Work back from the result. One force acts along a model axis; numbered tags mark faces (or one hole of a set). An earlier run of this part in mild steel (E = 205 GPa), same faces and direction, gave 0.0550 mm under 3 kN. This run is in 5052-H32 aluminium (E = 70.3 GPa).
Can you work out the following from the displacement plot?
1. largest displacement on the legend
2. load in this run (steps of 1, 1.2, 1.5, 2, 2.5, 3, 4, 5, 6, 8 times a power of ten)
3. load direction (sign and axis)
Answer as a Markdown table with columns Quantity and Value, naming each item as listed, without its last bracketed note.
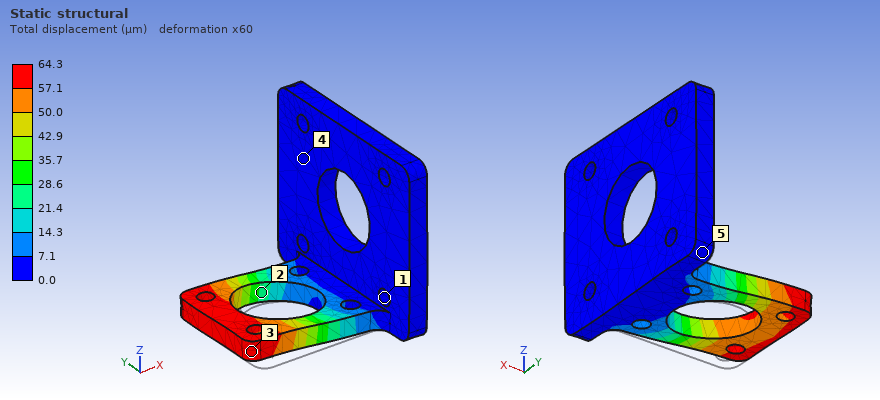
| Quantity | Value |
|---|---|
| largest displacement on the legend | 64.3 µm |
| load in this run | 1.2 kN |
| load direction | +Y |
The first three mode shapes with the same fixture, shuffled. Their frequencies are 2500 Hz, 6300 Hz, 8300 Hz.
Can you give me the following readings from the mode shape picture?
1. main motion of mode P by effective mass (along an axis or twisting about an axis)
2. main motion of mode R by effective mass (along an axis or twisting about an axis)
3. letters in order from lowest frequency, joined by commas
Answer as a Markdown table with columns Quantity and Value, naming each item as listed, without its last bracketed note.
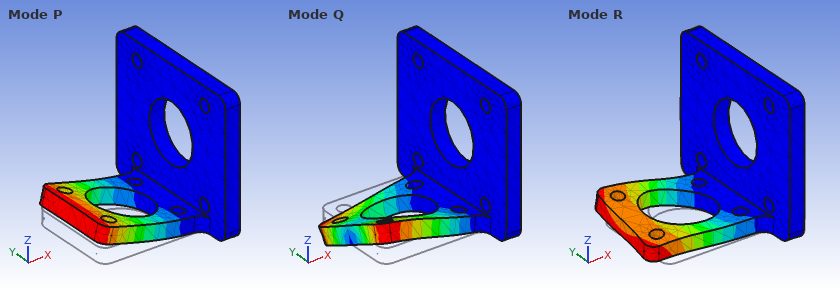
| Quantity | Value |
|---|---|
| main motion of mode P by effective mass | along Z |
| main motion of mode R by effective mass | along Y |
| letters in order from lowest frequency, joined by commas | P, Q, R |
